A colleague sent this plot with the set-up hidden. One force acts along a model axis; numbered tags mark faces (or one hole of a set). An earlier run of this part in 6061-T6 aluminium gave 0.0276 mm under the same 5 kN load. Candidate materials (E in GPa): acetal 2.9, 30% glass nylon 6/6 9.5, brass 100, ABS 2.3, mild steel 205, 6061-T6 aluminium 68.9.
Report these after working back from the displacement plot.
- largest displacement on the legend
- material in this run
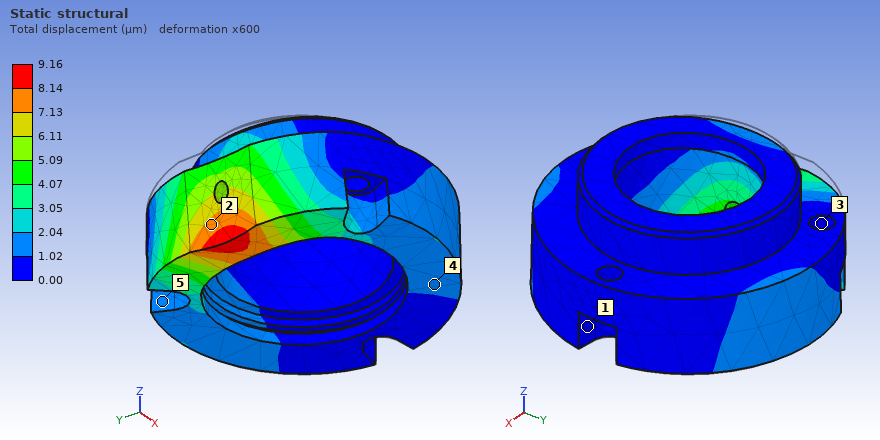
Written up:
9.16 µm
mild steel
